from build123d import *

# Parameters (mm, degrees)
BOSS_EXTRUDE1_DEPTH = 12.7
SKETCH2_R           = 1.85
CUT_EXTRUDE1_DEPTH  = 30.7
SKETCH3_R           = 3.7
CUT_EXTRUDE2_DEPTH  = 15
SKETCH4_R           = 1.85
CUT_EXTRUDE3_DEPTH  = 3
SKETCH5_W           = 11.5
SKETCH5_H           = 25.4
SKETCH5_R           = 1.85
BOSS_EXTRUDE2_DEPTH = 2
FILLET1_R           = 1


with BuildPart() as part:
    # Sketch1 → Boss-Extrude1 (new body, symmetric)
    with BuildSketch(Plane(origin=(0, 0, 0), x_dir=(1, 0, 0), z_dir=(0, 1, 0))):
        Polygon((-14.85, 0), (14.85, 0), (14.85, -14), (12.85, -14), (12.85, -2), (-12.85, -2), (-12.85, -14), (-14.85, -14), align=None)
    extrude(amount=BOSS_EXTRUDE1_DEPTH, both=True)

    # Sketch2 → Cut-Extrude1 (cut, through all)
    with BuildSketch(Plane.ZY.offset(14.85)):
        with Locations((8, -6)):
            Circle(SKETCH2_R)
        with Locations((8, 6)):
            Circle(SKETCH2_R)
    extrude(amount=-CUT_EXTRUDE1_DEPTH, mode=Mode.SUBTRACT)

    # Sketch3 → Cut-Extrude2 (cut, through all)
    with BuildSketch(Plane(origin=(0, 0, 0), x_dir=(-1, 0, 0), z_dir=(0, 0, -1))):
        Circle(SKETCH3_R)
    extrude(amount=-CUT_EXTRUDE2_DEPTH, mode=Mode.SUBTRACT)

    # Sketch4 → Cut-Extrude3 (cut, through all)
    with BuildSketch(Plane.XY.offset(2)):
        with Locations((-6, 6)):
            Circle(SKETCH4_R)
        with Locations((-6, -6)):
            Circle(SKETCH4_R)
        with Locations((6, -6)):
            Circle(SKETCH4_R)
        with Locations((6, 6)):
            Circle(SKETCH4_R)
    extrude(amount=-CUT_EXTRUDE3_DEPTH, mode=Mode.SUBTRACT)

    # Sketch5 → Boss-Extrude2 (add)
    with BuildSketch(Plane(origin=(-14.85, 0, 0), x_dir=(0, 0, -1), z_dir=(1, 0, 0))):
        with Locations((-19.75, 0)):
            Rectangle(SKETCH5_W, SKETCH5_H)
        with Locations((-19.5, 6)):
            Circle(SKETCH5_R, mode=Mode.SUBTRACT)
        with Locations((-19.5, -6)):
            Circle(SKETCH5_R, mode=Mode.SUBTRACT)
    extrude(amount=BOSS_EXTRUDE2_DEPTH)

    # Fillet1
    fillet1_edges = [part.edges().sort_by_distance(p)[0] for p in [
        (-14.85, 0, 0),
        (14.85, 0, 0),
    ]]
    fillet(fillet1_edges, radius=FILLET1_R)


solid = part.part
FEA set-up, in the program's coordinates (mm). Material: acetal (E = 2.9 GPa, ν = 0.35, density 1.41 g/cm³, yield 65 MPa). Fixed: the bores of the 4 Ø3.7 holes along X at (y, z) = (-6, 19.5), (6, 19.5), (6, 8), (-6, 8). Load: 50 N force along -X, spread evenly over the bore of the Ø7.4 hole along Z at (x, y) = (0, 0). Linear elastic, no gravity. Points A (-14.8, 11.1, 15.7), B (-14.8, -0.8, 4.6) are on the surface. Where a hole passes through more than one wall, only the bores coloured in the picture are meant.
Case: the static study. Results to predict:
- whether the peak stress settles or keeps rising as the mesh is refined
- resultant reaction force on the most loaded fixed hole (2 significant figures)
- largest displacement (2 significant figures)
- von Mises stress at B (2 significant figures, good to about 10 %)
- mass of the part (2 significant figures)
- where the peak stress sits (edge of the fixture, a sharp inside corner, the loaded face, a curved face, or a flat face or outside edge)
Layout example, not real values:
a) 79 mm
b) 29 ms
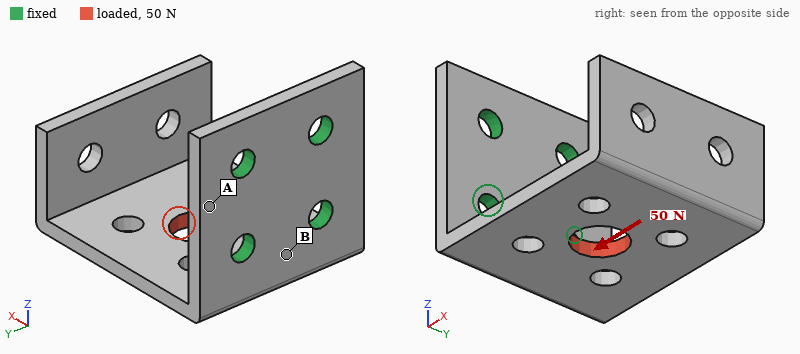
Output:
a) keeps rising
b) 27 N
c) 0.54 mm
d) 7.4 MPa
e) 4.2 g
f) edge of the fixture
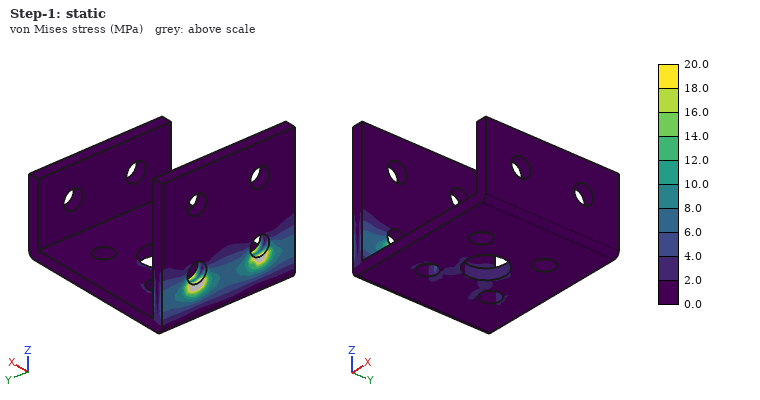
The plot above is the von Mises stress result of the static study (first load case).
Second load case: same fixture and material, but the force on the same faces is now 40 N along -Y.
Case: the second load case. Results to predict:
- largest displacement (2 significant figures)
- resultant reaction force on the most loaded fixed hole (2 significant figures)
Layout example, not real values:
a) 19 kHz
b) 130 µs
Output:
a) 0.52 mm
b) 46 N
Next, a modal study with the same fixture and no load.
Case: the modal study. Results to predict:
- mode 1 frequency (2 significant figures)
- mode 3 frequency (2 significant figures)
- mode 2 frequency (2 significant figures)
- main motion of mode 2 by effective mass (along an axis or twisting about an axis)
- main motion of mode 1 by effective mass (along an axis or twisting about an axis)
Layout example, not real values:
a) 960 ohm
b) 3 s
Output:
a) 270 Hz
b) 1200 Hz
c) 620 Hz
d) along Y
e) along Z
